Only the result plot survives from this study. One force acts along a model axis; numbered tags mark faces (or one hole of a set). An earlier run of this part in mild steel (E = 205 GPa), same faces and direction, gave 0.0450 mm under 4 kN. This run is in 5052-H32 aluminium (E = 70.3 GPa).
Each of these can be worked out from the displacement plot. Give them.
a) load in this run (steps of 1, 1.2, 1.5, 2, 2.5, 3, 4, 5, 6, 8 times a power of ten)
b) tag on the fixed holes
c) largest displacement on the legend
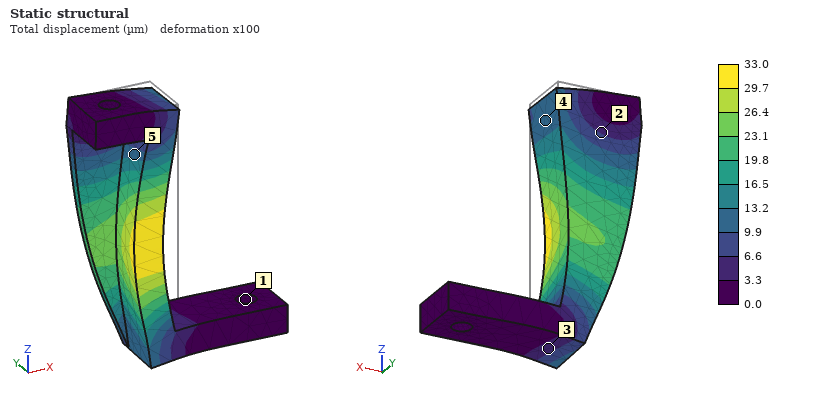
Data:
1 kN
1
33.0 µm
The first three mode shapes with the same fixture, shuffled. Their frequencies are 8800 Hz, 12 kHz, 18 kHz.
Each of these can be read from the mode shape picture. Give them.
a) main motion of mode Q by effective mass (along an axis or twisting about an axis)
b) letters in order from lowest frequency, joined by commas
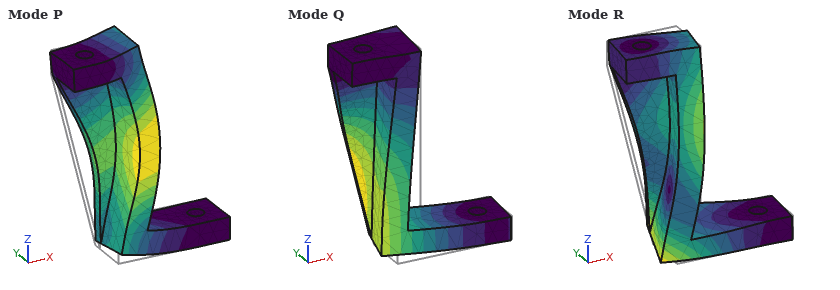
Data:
along Y
Q, P, R
